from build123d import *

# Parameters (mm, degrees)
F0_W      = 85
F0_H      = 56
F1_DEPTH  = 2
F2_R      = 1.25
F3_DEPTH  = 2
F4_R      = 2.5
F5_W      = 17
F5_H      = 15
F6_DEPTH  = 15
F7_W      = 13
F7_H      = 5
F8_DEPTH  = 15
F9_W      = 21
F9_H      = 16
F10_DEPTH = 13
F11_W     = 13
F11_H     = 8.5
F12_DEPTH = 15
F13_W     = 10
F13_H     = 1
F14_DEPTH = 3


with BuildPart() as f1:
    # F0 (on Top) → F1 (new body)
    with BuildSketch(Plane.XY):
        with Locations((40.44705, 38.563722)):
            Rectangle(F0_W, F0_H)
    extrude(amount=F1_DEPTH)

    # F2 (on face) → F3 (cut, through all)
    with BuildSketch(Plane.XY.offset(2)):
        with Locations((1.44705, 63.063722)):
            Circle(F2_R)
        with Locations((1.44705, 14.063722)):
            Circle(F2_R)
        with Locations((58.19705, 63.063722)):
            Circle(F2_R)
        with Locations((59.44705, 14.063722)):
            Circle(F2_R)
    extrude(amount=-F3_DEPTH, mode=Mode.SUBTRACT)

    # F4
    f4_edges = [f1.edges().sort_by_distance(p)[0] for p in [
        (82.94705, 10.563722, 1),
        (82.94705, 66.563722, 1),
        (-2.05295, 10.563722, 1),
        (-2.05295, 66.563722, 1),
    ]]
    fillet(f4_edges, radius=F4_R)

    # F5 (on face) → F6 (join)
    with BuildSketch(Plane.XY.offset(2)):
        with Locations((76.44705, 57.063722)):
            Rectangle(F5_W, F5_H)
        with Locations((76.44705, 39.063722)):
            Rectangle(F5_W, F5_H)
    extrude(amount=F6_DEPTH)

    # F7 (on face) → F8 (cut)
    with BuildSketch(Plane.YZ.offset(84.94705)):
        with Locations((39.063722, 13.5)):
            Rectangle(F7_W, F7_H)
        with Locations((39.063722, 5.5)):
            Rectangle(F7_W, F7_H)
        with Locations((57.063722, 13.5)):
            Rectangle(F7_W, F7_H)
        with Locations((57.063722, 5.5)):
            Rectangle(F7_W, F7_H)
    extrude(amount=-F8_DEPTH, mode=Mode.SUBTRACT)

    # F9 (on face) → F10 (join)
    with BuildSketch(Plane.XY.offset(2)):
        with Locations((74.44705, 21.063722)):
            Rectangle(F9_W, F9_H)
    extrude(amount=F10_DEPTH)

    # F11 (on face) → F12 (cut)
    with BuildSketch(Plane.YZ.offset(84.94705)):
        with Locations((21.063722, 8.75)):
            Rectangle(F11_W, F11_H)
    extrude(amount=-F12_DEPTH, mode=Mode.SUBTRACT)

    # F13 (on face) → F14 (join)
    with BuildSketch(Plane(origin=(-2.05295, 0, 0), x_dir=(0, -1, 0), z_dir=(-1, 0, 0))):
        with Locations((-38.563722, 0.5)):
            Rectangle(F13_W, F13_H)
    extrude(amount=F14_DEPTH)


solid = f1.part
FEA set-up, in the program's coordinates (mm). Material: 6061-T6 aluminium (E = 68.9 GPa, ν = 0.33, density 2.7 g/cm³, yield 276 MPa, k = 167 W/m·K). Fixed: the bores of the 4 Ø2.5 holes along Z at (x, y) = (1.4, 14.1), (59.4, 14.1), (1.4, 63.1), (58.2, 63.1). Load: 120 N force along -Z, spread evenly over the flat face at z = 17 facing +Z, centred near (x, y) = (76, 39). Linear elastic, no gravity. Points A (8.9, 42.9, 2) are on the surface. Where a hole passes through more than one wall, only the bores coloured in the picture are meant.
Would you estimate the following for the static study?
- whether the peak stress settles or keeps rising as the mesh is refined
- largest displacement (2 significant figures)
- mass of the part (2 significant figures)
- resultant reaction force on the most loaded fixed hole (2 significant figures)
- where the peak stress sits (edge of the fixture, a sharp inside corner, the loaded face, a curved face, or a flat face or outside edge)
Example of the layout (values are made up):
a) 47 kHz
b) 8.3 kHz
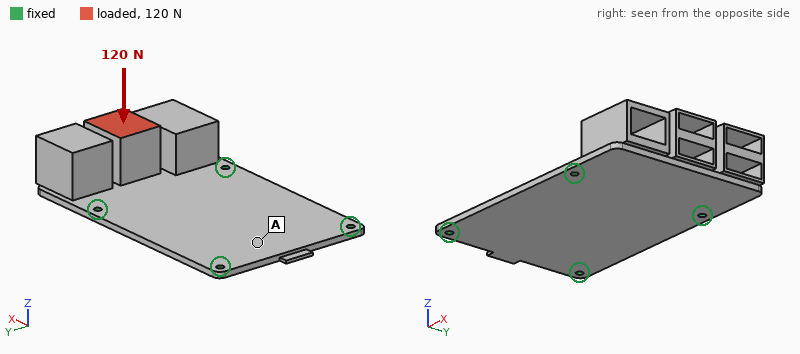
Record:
a) keeps rising
b) 0.26 mm
c) 43 g
d) 67 N
e) edge of the fixture
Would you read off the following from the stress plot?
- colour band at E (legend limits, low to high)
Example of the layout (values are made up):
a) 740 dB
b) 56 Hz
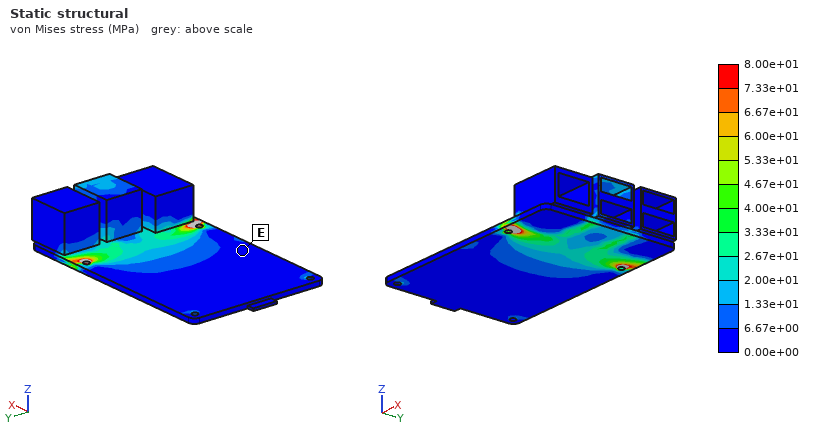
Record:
a) 0.00e+00 to 6.67e+00 MPa
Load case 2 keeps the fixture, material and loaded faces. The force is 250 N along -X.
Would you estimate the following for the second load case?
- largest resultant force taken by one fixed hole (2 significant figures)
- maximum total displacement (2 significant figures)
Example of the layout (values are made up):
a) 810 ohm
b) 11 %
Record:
a) 100 N
b) 0.50 mm
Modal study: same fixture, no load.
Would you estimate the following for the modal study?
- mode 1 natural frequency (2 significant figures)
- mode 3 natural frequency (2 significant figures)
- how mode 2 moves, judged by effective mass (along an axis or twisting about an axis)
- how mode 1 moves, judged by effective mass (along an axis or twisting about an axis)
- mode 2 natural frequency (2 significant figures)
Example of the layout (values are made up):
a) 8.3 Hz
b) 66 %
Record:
a) 980 Hz
b) 3100 Hz
c) along Z
d) along Z
e) 2300 Hz
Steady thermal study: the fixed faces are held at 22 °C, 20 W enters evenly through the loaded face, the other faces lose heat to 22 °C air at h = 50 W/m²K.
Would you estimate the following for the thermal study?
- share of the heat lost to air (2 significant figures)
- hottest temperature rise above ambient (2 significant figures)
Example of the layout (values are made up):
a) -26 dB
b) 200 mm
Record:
a) 40 %
b) 54 K
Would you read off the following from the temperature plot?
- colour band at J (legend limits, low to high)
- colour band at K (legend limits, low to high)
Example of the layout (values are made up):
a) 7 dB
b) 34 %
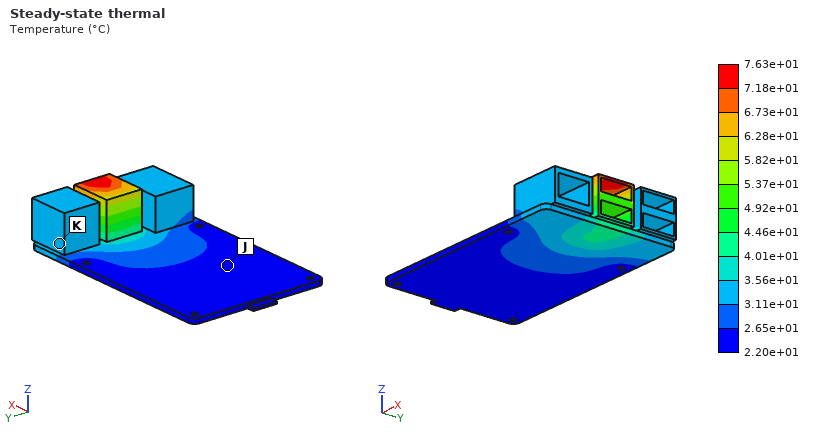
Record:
a) 2.20e+01 to 2.65e+01 °C
b) 3.11e+01 to 3.56e+01 °C
